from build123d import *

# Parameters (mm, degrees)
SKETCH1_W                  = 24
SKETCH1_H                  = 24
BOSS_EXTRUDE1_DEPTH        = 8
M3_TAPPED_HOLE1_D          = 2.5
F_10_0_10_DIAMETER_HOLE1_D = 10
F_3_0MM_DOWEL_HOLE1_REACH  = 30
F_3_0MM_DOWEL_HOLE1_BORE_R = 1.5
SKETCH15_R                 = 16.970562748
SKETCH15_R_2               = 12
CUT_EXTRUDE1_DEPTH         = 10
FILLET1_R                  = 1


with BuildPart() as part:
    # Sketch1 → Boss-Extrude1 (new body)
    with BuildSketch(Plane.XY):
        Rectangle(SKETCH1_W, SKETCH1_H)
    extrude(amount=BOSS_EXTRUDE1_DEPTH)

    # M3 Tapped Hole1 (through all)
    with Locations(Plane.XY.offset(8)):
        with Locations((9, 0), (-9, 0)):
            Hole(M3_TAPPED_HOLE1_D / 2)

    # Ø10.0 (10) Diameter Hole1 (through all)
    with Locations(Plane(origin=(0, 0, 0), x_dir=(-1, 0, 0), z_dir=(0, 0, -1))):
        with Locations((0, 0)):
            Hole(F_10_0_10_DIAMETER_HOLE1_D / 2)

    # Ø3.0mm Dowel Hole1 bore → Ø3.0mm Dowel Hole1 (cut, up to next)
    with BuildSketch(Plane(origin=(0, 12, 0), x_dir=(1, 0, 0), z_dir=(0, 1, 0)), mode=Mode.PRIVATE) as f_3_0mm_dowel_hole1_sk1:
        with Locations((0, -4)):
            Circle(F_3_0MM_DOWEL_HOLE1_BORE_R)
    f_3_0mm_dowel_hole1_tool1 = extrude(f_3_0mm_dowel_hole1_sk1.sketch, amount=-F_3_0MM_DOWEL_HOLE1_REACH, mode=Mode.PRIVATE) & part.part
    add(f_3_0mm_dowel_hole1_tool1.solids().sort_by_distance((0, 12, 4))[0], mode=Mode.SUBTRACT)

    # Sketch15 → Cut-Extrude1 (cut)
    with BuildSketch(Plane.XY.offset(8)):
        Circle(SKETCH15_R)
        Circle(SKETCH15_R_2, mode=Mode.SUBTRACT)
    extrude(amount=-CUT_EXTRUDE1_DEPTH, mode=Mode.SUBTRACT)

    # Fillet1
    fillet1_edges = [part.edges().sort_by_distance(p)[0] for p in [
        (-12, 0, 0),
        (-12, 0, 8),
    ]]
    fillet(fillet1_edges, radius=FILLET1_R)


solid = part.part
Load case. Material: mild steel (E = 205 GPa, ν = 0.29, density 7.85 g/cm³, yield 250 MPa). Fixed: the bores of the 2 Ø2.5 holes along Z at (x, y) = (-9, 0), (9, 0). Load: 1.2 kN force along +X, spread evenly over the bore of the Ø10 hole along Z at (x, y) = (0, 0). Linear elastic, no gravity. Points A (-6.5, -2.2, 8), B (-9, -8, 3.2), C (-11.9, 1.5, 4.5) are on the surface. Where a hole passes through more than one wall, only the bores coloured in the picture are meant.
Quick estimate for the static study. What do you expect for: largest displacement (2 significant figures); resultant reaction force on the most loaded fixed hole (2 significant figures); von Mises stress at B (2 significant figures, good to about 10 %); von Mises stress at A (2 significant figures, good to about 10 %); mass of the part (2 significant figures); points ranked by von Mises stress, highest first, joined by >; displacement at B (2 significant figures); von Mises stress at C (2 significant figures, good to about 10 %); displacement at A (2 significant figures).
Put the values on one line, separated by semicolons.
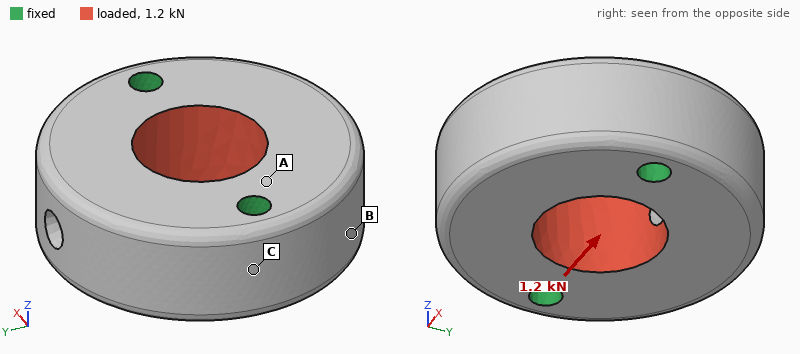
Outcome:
0.51 µm; 600 N; 2.7 MPa; 11 MPa; 22 g; A > C > B; 0.38 µm; 7.2 MPa; 0.19 µm
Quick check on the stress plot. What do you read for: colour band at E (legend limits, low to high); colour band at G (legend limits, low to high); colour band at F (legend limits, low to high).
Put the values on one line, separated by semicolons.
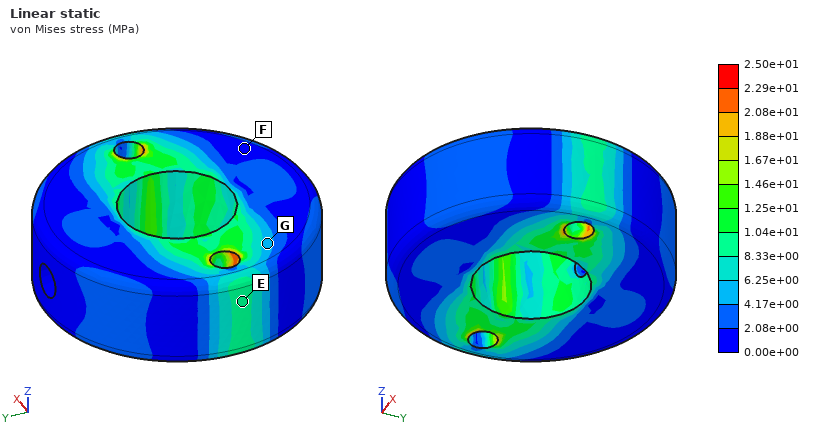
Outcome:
8.33e+00 to 1.04e+01 MPa; 4.17e+00 to 6.25e+00 MPa; 0.00e+00 to 2.08e+00 MPa
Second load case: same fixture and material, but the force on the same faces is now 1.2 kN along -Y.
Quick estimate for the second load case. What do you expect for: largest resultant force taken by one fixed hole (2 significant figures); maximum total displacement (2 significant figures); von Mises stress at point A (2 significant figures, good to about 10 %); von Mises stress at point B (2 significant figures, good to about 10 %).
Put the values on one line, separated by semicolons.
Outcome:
600 N; 0.50 µm; 10 MPa; 3.4 MPa
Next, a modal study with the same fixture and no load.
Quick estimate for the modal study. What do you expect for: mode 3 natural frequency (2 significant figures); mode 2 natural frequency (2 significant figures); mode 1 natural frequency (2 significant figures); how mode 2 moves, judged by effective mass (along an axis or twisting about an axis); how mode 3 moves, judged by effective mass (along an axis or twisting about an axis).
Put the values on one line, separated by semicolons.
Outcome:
51 kHz; 36 kHz; 33 kHz; along Z; twisting about Z
